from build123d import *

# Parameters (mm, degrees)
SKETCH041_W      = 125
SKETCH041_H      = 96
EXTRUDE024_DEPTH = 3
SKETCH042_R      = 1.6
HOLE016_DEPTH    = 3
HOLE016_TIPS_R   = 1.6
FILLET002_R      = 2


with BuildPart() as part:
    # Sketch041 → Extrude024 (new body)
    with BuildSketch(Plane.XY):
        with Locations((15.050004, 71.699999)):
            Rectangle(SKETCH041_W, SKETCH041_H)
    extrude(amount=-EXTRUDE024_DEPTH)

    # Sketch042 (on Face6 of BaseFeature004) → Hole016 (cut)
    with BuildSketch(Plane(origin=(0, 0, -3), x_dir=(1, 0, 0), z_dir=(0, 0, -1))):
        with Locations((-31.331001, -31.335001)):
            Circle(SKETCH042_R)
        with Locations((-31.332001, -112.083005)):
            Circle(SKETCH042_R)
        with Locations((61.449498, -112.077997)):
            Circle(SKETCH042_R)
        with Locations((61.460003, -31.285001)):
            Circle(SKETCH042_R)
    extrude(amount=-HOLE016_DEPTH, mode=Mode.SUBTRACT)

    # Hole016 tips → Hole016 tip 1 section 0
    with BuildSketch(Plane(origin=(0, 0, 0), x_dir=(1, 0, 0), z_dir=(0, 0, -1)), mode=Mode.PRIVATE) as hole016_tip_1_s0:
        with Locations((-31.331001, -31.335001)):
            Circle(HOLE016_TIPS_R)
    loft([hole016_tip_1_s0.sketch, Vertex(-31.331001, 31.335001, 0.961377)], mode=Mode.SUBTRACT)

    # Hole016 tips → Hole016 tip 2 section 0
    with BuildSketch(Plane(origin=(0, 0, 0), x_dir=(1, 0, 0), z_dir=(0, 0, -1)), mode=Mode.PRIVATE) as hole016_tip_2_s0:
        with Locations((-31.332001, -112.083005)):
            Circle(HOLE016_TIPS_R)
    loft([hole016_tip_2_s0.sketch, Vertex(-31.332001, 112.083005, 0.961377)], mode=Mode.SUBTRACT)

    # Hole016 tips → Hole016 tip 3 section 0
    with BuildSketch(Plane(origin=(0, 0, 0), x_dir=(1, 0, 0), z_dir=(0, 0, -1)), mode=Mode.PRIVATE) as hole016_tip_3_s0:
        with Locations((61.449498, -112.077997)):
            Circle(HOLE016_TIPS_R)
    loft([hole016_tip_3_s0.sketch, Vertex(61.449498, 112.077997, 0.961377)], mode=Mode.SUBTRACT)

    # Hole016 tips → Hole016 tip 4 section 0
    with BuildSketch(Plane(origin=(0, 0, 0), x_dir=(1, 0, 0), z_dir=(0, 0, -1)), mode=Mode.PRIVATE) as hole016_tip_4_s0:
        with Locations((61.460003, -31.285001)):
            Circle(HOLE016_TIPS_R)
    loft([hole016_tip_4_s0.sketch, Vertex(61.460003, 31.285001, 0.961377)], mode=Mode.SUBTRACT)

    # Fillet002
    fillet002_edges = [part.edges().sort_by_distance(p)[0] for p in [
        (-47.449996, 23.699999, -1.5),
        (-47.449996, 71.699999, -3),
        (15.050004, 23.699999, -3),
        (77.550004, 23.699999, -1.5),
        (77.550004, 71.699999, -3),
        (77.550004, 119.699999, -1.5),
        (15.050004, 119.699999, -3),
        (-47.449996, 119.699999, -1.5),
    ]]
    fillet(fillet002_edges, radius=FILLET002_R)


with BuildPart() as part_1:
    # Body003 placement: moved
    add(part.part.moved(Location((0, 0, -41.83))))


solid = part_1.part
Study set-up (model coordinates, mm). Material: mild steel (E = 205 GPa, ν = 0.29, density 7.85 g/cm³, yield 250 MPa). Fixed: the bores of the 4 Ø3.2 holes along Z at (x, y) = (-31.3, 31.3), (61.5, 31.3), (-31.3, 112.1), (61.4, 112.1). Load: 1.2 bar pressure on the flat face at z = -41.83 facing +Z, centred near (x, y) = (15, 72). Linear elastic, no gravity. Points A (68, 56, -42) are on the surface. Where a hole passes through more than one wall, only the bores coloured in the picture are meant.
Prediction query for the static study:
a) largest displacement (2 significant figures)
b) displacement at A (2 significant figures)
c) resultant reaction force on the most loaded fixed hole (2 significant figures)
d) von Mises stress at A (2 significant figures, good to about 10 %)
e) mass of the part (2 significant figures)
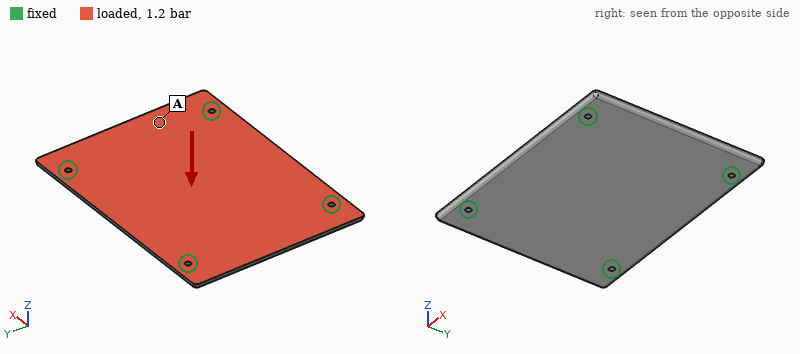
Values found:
0.11 mm
0.029 mm
360 N
21 MPa
280 g
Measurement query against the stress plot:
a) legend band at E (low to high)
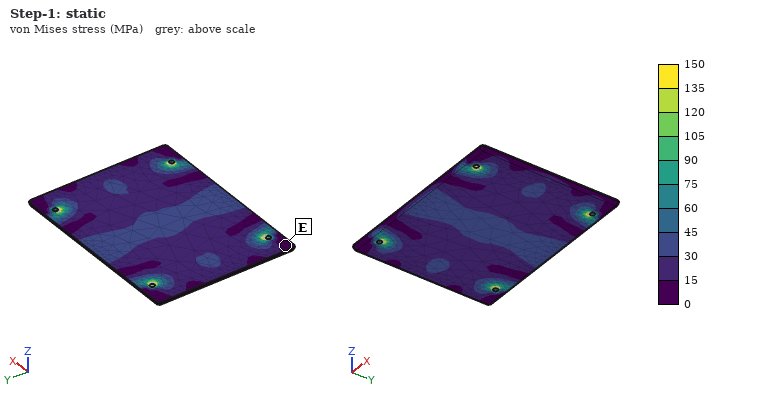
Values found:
0 to 15 MPa
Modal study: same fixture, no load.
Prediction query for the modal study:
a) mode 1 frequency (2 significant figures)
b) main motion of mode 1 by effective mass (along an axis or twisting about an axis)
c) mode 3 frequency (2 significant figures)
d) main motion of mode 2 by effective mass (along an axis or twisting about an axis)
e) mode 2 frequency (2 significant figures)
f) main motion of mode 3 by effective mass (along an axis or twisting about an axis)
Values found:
1300 Hz
along Z
2300 Hz
twisting about X
2100 Hz
twisting about Y
